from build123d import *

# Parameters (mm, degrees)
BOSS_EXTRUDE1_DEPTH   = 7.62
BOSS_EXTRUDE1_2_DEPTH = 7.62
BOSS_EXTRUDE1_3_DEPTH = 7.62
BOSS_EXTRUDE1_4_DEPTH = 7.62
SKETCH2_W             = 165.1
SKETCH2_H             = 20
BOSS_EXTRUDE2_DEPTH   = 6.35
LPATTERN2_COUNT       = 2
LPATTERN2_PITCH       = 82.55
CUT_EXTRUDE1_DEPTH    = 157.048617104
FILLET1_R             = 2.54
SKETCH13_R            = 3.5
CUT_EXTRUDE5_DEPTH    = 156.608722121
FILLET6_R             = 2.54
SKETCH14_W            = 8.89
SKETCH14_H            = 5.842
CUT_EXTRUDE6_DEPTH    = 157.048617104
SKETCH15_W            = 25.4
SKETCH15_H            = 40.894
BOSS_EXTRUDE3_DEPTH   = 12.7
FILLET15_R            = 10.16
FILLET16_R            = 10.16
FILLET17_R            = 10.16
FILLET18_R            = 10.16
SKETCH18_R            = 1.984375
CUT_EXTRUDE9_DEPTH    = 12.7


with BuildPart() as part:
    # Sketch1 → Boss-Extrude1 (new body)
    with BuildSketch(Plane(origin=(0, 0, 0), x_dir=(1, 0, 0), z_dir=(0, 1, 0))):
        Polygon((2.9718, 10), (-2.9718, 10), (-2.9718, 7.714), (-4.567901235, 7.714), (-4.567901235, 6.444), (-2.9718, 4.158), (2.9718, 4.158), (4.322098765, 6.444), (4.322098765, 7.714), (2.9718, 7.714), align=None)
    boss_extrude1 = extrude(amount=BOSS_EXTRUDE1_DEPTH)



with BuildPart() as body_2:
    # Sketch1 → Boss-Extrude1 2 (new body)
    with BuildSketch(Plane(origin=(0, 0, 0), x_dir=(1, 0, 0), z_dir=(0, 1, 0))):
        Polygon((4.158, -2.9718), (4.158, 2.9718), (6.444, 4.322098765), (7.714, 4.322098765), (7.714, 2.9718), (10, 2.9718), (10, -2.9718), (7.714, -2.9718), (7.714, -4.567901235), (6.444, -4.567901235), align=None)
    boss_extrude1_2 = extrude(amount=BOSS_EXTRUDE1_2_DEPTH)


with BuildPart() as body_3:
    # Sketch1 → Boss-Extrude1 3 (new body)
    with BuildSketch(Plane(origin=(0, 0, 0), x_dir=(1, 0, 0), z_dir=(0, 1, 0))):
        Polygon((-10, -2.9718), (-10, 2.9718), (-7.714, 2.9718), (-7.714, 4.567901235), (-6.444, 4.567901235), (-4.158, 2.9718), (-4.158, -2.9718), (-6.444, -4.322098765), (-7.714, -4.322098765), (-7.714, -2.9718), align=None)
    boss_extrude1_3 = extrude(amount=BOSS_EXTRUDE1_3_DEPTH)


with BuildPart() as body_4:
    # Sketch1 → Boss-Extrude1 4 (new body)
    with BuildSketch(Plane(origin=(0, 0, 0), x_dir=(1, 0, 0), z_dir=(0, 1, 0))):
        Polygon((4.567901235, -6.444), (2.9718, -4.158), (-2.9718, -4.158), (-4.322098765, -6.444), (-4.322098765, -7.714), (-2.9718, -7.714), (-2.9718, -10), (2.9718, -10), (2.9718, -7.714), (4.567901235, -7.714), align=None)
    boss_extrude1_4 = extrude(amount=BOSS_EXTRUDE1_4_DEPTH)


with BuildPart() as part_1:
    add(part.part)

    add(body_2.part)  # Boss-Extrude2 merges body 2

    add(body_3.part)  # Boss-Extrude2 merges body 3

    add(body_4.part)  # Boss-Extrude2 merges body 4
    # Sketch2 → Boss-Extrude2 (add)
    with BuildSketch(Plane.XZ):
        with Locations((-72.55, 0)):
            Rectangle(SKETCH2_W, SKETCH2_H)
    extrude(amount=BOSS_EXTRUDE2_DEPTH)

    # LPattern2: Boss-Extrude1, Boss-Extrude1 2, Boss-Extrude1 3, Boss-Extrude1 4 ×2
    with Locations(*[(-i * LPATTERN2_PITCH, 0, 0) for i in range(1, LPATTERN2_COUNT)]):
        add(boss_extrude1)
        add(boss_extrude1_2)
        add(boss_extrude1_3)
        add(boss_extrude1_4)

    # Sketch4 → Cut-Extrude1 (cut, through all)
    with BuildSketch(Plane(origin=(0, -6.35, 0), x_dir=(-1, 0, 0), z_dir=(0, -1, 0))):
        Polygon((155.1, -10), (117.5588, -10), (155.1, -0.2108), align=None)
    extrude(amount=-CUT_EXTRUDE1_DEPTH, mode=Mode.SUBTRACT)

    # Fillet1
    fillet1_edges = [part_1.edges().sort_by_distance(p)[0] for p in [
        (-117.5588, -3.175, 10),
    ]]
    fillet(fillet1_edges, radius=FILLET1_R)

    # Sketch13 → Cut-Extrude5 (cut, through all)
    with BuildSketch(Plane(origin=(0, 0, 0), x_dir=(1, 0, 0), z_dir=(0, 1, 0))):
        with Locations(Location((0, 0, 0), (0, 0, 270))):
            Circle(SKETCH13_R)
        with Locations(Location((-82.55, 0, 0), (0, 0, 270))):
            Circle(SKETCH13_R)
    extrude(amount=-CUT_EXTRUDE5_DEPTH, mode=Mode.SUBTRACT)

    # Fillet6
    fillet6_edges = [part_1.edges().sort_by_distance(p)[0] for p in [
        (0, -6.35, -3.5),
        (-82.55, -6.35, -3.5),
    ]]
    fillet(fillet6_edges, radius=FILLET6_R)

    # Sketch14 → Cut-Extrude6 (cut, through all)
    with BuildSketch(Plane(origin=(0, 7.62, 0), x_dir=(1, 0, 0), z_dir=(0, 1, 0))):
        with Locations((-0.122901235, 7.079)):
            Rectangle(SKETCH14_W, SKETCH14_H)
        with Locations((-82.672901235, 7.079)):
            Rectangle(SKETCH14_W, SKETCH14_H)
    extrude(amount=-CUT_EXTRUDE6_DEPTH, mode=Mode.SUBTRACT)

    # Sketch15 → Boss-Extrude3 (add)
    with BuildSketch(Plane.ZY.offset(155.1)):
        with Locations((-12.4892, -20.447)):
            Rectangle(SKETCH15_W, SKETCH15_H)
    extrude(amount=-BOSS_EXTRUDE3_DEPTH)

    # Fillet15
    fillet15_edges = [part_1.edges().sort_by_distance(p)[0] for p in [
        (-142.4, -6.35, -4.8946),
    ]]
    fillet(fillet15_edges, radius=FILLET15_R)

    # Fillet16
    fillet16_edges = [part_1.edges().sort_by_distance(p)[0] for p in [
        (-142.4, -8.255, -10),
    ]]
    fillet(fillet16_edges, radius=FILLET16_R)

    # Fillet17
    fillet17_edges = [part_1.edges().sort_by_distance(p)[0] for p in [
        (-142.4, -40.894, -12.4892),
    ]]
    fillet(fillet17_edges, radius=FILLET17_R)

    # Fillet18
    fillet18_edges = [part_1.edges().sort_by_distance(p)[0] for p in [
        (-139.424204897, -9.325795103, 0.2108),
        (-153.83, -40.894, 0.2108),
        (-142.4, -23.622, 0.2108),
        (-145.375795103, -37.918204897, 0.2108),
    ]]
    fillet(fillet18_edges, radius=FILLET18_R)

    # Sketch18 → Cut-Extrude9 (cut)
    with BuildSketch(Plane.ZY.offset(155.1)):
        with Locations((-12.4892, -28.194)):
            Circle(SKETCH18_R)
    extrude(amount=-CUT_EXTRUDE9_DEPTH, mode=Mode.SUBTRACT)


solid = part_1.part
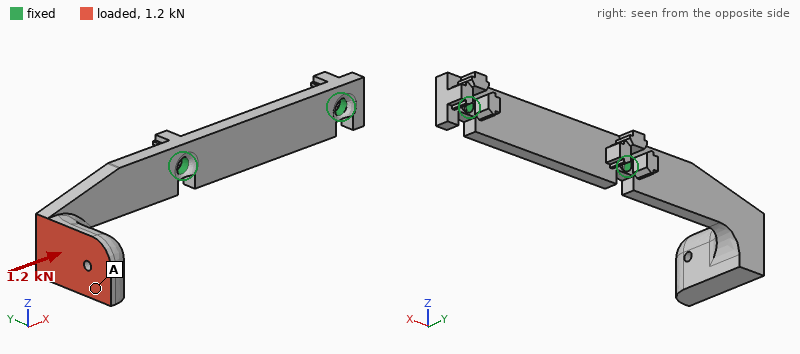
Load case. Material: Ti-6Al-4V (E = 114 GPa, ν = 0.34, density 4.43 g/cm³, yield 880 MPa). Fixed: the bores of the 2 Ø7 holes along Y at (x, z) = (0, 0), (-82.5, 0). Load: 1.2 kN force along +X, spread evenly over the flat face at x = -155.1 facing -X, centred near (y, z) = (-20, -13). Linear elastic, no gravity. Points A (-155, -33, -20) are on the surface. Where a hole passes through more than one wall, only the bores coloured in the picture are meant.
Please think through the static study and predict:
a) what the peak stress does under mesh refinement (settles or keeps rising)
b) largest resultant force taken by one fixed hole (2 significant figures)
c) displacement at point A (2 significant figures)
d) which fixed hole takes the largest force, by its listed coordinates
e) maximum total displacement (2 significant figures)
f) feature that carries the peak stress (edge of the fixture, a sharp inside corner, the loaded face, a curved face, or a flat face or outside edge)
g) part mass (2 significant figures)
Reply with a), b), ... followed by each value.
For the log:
a) keeps rising
b) 1.2 kN
c) 1.5 mm
d) (-82.5, 0)
e) 1.7 mm
f) edge of the fixture
g) 140 g
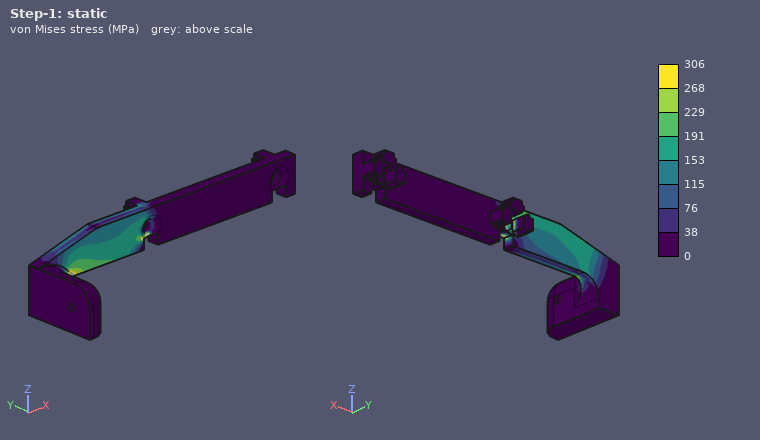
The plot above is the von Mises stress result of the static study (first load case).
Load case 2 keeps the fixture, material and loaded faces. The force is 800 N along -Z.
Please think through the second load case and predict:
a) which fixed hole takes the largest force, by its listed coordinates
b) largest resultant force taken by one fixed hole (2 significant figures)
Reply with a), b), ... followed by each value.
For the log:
a) (-82.5, 0)
b) 1.1 kN
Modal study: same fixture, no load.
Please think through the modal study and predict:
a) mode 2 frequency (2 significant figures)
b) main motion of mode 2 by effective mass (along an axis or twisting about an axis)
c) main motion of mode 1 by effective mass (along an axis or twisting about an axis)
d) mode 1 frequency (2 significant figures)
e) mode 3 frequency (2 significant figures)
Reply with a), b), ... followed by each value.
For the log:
a) 750 Hz
b) along Z
c) along Y
d) 390 Hz
e) 1800 Hz
